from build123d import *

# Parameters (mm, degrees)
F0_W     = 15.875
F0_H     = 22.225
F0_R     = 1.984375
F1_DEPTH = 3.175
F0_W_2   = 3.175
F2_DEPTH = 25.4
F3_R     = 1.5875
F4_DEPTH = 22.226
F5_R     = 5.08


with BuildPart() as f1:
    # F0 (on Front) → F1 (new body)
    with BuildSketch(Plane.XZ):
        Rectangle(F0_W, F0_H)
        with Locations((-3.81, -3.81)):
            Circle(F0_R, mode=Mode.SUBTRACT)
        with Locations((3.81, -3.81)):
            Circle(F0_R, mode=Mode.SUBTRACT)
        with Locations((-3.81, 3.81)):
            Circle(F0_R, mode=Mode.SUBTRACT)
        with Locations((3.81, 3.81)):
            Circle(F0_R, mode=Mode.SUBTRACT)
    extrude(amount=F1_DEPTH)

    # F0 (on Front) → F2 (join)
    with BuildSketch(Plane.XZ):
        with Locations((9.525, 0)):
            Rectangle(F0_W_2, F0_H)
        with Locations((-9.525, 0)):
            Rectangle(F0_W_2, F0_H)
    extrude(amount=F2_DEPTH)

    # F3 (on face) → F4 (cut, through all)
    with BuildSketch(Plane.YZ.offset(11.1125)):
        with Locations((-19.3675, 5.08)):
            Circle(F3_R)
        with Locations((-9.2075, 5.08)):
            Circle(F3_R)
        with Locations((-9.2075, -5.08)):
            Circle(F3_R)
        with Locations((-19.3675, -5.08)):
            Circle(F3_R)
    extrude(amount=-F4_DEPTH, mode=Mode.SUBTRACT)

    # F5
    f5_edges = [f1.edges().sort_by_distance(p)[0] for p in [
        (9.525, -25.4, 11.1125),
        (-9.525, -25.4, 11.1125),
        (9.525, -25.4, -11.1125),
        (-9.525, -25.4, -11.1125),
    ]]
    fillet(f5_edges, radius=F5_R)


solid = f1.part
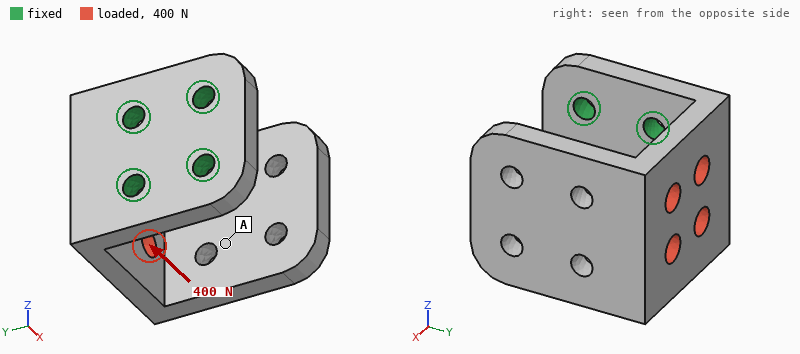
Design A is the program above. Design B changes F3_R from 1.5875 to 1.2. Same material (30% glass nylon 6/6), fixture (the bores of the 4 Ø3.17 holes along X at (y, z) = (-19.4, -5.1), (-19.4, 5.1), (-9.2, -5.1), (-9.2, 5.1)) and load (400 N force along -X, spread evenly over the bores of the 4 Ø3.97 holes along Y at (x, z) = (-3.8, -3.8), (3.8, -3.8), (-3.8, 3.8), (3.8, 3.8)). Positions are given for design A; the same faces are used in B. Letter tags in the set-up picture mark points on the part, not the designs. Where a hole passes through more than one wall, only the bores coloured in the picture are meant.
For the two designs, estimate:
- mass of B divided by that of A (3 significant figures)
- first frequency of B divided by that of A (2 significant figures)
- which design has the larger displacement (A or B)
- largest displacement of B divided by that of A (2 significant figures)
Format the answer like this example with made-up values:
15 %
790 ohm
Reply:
1.02
0.98
B
1.1
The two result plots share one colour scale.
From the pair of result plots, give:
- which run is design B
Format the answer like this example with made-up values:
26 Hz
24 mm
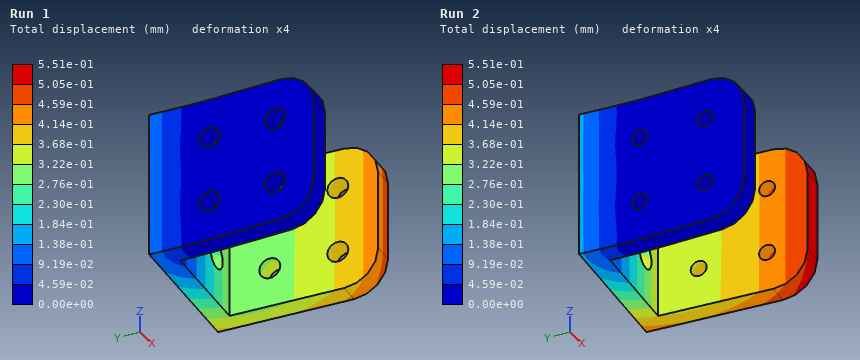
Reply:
Run 2
